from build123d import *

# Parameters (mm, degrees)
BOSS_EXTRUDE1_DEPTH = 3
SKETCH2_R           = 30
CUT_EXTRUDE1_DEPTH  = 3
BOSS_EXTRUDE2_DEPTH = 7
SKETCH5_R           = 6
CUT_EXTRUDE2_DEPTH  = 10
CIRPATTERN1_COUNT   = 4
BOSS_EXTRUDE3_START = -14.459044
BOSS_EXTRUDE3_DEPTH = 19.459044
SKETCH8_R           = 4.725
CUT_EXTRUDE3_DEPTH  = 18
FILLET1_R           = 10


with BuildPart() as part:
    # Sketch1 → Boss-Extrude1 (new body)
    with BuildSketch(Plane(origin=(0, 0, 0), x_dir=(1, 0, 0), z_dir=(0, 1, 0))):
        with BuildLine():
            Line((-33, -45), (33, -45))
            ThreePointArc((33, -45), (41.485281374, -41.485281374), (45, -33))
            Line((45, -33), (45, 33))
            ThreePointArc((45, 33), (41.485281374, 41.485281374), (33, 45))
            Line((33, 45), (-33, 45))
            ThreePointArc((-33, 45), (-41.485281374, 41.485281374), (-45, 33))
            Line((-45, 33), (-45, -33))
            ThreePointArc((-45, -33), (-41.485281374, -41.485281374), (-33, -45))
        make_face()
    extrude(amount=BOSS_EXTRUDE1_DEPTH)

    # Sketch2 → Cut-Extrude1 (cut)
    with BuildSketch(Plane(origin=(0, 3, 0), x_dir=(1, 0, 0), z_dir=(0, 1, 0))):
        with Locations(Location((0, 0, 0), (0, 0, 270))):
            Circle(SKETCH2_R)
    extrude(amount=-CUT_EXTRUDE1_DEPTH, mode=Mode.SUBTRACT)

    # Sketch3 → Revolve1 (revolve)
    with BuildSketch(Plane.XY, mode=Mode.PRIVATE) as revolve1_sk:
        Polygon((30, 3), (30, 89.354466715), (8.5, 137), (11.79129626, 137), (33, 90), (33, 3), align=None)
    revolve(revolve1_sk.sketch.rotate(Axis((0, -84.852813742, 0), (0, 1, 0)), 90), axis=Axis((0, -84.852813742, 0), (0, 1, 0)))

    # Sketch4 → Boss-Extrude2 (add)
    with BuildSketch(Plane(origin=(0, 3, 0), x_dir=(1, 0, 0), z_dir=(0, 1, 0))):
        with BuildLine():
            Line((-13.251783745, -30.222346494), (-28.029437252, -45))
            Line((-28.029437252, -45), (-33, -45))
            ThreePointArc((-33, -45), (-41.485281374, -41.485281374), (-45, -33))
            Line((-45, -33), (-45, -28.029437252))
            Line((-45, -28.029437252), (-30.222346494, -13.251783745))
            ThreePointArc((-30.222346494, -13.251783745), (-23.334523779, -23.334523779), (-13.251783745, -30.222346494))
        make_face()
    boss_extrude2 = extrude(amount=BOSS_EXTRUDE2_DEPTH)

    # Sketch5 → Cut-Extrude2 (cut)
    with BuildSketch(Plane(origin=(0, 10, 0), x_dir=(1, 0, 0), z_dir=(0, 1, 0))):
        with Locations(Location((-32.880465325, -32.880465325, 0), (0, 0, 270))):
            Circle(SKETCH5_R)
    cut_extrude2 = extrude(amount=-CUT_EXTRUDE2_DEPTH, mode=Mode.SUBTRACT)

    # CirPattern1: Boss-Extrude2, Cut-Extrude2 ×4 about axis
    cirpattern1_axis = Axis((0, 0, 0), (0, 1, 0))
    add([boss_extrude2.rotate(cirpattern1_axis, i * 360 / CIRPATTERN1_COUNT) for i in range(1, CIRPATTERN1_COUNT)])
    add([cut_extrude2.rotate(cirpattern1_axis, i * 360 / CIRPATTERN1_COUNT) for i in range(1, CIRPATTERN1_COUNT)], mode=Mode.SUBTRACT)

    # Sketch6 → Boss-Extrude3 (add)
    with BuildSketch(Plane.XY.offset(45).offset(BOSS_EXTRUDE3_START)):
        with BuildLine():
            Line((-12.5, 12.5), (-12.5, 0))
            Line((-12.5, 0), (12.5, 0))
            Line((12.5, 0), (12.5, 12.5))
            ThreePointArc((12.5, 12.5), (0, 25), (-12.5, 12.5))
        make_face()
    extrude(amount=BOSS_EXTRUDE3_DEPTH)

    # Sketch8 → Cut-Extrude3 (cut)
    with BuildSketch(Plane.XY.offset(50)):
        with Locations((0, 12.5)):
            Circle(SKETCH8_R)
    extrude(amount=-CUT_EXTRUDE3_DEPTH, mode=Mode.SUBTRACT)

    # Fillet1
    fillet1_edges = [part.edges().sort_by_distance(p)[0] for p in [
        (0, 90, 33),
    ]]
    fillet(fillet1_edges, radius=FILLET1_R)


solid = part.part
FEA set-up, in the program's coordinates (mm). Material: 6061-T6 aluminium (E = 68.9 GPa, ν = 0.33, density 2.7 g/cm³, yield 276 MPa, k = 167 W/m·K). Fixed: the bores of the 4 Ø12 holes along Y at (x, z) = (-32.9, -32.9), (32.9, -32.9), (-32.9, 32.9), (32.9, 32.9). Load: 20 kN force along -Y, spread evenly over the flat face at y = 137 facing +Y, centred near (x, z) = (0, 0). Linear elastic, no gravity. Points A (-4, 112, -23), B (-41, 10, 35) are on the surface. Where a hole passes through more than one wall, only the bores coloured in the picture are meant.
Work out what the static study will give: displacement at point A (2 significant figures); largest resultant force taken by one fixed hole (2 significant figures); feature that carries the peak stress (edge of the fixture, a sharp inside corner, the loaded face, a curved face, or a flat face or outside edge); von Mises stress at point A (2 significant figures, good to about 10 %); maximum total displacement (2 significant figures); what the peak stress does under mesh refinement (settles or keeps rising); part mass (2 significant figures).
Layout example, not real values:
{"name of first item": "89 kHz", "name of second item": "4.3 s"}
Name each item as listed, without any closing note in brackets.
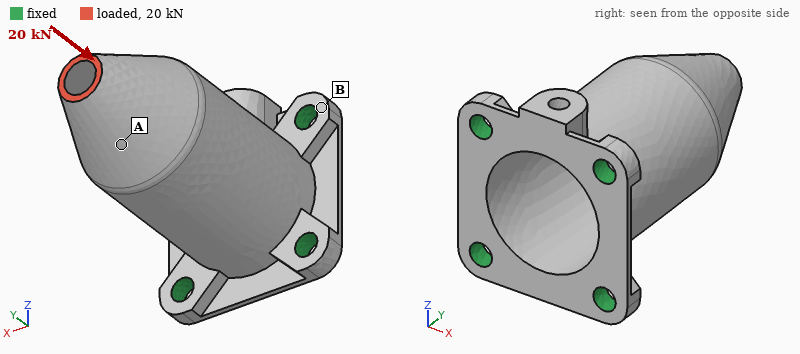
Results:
{"displacement at point A": "0.094 mm", "largest resultant force taken by one fixed hole": "5.1 kN", "feature that carries the peak stress": "a sharp inside corner", "von Mises stress at point A": "55 MPa", "maximum total displacement": "0.16 mm", "what the peak stress does under mesh refinement": "keeps rising", "part mass": "290 g"}
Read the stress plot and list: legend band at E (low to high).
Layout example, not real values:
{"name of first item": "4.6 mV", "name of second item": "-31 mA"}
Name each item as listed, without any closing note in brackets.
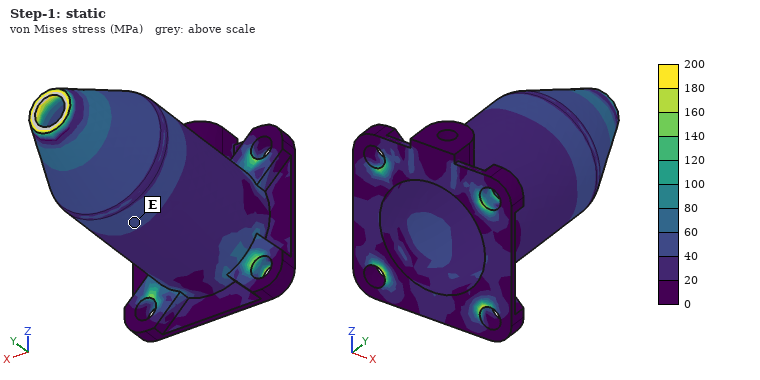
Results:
{"legend band at E": "40 to 60 MPa"}
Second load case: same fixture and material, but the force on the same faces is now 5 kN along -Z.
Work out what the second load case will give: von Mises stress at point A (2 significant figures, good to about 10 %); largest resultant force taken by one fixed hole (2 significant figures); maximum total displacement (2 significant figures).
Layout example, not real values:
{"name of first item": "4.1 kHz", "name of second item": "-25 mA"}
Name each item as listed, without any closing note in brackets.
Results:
{"von Mises stress at point A": "35 MPa", "largest resultant force taken by one fixed hole": "6.3 kN", "maximum total displacement": "0.48 mm"}
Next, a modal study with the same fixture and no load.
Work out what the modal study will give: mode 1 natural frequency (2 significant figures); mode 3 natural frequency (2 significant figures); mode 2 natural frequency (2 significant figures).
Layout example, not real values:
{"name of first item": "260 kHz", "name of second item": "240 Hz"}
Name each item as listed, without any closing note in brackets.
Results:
{"mode 1 natural frequency": "2300 Hz", "mode 3 natural frequency": "5000 Hz", "mode 2 natural frequency": "2300 Hz"}
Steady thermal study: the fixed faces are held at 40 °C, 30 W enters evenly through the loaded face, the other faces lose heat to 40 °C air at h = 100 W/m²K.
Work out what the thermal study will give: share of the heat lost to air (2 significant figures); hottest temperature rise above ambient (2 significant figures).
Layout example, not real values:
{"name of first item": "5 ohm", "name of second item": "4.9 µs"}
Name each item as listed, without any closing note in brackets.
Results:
{"share of the heat lost to air": "86 %", "hottest temperature rise above ambient": "27 K"}
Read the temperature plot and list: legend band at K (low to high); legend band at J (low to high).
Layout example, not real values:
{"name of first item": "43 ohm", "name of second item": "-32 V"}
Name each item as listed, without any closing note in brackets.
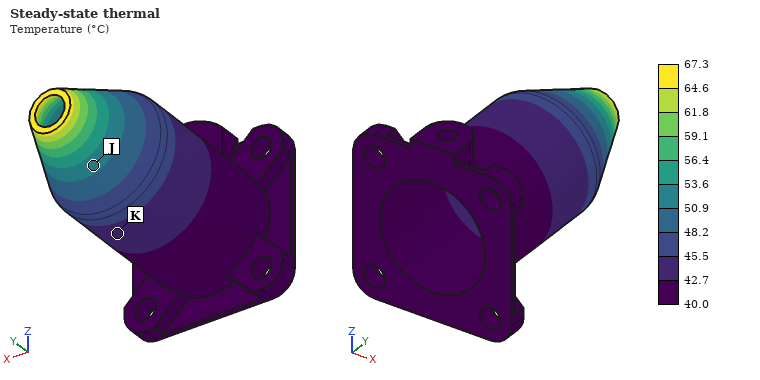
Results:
{"legend band at K": "42.7 to 45.5 °C", "legend band at J": "50.9 to 53.6 °C"}
